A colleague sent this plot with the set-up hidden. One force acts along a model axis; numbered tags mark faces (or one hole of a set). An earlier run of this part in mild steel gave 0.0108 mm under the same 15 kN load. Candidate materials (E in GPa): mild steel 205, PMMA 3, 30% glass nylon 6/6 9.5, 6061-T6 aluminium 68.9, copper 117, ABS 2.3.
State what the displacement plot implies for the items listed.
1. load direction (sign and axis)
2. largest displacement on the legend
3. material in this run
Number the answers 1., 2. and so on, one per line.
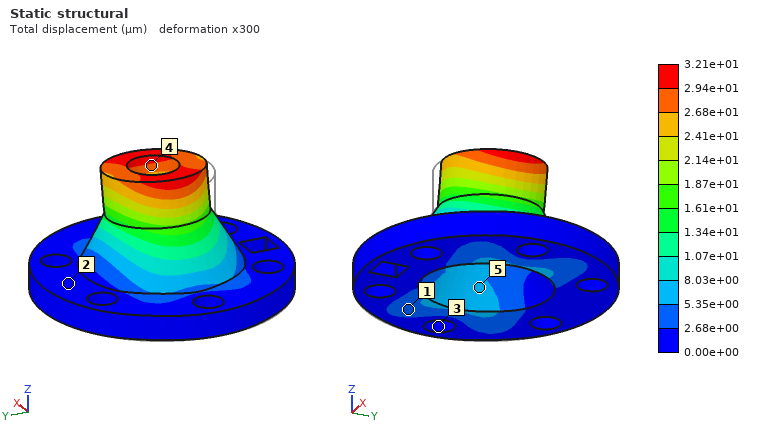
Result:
1. +X
2. 3.21e+01 µm
3. 6061-T6 aluminium
